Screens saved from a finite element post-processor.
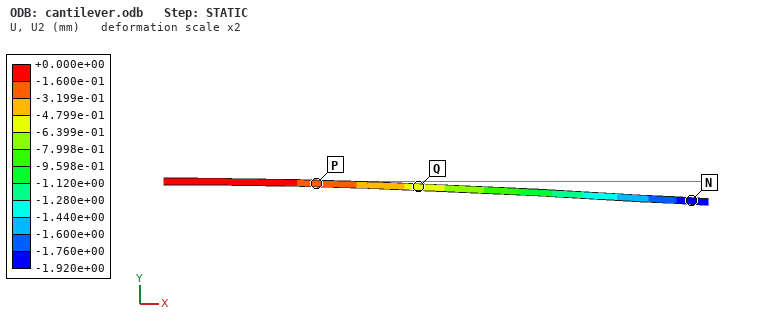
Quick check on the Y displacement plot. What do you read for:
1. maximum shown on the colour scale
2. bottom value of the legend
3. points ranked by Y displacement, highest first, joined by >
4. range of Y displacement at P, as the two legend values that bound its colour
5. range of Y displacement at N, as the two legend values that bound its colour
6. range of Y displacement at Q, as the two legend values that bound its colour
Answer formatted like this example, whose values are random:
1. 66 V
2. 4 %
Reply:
1. +0.000e+00 mm
2. -1.920e+00 mm
3. P > Q > N
4. -3.199e-01 to -1.600e-01 mm
5. -1.920e+00 to -1.760e+00 mm
6. -6.399e-01 to -4.799e-01 mm
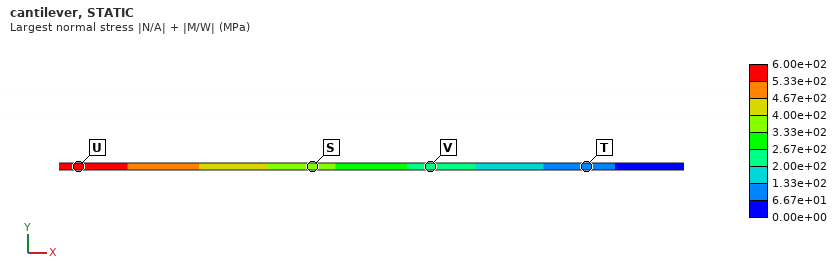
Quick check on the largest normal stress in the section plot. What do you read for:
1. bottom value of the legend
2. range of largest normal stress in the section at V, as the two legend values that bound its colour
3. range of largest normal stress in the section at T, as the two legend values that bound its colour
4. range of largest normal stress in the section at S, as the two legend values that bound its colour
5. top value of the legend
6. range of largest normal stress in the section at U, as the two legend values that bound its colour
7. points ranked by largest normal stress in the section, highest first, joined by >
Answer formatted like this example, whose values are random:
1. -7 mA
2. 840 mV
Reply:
1. 0.00e+00 MPa
2. 2.00e+02 to 2.67e+02 MPa
3. 6.67e+01 to 1.33e+02 MPa
4. 3.33e+02 to 4.00e+02 MPa
5. 6.00e+02 MPa
6. 5.33e+02 to 6.00e+02 MPa
7. U > S > V > T
